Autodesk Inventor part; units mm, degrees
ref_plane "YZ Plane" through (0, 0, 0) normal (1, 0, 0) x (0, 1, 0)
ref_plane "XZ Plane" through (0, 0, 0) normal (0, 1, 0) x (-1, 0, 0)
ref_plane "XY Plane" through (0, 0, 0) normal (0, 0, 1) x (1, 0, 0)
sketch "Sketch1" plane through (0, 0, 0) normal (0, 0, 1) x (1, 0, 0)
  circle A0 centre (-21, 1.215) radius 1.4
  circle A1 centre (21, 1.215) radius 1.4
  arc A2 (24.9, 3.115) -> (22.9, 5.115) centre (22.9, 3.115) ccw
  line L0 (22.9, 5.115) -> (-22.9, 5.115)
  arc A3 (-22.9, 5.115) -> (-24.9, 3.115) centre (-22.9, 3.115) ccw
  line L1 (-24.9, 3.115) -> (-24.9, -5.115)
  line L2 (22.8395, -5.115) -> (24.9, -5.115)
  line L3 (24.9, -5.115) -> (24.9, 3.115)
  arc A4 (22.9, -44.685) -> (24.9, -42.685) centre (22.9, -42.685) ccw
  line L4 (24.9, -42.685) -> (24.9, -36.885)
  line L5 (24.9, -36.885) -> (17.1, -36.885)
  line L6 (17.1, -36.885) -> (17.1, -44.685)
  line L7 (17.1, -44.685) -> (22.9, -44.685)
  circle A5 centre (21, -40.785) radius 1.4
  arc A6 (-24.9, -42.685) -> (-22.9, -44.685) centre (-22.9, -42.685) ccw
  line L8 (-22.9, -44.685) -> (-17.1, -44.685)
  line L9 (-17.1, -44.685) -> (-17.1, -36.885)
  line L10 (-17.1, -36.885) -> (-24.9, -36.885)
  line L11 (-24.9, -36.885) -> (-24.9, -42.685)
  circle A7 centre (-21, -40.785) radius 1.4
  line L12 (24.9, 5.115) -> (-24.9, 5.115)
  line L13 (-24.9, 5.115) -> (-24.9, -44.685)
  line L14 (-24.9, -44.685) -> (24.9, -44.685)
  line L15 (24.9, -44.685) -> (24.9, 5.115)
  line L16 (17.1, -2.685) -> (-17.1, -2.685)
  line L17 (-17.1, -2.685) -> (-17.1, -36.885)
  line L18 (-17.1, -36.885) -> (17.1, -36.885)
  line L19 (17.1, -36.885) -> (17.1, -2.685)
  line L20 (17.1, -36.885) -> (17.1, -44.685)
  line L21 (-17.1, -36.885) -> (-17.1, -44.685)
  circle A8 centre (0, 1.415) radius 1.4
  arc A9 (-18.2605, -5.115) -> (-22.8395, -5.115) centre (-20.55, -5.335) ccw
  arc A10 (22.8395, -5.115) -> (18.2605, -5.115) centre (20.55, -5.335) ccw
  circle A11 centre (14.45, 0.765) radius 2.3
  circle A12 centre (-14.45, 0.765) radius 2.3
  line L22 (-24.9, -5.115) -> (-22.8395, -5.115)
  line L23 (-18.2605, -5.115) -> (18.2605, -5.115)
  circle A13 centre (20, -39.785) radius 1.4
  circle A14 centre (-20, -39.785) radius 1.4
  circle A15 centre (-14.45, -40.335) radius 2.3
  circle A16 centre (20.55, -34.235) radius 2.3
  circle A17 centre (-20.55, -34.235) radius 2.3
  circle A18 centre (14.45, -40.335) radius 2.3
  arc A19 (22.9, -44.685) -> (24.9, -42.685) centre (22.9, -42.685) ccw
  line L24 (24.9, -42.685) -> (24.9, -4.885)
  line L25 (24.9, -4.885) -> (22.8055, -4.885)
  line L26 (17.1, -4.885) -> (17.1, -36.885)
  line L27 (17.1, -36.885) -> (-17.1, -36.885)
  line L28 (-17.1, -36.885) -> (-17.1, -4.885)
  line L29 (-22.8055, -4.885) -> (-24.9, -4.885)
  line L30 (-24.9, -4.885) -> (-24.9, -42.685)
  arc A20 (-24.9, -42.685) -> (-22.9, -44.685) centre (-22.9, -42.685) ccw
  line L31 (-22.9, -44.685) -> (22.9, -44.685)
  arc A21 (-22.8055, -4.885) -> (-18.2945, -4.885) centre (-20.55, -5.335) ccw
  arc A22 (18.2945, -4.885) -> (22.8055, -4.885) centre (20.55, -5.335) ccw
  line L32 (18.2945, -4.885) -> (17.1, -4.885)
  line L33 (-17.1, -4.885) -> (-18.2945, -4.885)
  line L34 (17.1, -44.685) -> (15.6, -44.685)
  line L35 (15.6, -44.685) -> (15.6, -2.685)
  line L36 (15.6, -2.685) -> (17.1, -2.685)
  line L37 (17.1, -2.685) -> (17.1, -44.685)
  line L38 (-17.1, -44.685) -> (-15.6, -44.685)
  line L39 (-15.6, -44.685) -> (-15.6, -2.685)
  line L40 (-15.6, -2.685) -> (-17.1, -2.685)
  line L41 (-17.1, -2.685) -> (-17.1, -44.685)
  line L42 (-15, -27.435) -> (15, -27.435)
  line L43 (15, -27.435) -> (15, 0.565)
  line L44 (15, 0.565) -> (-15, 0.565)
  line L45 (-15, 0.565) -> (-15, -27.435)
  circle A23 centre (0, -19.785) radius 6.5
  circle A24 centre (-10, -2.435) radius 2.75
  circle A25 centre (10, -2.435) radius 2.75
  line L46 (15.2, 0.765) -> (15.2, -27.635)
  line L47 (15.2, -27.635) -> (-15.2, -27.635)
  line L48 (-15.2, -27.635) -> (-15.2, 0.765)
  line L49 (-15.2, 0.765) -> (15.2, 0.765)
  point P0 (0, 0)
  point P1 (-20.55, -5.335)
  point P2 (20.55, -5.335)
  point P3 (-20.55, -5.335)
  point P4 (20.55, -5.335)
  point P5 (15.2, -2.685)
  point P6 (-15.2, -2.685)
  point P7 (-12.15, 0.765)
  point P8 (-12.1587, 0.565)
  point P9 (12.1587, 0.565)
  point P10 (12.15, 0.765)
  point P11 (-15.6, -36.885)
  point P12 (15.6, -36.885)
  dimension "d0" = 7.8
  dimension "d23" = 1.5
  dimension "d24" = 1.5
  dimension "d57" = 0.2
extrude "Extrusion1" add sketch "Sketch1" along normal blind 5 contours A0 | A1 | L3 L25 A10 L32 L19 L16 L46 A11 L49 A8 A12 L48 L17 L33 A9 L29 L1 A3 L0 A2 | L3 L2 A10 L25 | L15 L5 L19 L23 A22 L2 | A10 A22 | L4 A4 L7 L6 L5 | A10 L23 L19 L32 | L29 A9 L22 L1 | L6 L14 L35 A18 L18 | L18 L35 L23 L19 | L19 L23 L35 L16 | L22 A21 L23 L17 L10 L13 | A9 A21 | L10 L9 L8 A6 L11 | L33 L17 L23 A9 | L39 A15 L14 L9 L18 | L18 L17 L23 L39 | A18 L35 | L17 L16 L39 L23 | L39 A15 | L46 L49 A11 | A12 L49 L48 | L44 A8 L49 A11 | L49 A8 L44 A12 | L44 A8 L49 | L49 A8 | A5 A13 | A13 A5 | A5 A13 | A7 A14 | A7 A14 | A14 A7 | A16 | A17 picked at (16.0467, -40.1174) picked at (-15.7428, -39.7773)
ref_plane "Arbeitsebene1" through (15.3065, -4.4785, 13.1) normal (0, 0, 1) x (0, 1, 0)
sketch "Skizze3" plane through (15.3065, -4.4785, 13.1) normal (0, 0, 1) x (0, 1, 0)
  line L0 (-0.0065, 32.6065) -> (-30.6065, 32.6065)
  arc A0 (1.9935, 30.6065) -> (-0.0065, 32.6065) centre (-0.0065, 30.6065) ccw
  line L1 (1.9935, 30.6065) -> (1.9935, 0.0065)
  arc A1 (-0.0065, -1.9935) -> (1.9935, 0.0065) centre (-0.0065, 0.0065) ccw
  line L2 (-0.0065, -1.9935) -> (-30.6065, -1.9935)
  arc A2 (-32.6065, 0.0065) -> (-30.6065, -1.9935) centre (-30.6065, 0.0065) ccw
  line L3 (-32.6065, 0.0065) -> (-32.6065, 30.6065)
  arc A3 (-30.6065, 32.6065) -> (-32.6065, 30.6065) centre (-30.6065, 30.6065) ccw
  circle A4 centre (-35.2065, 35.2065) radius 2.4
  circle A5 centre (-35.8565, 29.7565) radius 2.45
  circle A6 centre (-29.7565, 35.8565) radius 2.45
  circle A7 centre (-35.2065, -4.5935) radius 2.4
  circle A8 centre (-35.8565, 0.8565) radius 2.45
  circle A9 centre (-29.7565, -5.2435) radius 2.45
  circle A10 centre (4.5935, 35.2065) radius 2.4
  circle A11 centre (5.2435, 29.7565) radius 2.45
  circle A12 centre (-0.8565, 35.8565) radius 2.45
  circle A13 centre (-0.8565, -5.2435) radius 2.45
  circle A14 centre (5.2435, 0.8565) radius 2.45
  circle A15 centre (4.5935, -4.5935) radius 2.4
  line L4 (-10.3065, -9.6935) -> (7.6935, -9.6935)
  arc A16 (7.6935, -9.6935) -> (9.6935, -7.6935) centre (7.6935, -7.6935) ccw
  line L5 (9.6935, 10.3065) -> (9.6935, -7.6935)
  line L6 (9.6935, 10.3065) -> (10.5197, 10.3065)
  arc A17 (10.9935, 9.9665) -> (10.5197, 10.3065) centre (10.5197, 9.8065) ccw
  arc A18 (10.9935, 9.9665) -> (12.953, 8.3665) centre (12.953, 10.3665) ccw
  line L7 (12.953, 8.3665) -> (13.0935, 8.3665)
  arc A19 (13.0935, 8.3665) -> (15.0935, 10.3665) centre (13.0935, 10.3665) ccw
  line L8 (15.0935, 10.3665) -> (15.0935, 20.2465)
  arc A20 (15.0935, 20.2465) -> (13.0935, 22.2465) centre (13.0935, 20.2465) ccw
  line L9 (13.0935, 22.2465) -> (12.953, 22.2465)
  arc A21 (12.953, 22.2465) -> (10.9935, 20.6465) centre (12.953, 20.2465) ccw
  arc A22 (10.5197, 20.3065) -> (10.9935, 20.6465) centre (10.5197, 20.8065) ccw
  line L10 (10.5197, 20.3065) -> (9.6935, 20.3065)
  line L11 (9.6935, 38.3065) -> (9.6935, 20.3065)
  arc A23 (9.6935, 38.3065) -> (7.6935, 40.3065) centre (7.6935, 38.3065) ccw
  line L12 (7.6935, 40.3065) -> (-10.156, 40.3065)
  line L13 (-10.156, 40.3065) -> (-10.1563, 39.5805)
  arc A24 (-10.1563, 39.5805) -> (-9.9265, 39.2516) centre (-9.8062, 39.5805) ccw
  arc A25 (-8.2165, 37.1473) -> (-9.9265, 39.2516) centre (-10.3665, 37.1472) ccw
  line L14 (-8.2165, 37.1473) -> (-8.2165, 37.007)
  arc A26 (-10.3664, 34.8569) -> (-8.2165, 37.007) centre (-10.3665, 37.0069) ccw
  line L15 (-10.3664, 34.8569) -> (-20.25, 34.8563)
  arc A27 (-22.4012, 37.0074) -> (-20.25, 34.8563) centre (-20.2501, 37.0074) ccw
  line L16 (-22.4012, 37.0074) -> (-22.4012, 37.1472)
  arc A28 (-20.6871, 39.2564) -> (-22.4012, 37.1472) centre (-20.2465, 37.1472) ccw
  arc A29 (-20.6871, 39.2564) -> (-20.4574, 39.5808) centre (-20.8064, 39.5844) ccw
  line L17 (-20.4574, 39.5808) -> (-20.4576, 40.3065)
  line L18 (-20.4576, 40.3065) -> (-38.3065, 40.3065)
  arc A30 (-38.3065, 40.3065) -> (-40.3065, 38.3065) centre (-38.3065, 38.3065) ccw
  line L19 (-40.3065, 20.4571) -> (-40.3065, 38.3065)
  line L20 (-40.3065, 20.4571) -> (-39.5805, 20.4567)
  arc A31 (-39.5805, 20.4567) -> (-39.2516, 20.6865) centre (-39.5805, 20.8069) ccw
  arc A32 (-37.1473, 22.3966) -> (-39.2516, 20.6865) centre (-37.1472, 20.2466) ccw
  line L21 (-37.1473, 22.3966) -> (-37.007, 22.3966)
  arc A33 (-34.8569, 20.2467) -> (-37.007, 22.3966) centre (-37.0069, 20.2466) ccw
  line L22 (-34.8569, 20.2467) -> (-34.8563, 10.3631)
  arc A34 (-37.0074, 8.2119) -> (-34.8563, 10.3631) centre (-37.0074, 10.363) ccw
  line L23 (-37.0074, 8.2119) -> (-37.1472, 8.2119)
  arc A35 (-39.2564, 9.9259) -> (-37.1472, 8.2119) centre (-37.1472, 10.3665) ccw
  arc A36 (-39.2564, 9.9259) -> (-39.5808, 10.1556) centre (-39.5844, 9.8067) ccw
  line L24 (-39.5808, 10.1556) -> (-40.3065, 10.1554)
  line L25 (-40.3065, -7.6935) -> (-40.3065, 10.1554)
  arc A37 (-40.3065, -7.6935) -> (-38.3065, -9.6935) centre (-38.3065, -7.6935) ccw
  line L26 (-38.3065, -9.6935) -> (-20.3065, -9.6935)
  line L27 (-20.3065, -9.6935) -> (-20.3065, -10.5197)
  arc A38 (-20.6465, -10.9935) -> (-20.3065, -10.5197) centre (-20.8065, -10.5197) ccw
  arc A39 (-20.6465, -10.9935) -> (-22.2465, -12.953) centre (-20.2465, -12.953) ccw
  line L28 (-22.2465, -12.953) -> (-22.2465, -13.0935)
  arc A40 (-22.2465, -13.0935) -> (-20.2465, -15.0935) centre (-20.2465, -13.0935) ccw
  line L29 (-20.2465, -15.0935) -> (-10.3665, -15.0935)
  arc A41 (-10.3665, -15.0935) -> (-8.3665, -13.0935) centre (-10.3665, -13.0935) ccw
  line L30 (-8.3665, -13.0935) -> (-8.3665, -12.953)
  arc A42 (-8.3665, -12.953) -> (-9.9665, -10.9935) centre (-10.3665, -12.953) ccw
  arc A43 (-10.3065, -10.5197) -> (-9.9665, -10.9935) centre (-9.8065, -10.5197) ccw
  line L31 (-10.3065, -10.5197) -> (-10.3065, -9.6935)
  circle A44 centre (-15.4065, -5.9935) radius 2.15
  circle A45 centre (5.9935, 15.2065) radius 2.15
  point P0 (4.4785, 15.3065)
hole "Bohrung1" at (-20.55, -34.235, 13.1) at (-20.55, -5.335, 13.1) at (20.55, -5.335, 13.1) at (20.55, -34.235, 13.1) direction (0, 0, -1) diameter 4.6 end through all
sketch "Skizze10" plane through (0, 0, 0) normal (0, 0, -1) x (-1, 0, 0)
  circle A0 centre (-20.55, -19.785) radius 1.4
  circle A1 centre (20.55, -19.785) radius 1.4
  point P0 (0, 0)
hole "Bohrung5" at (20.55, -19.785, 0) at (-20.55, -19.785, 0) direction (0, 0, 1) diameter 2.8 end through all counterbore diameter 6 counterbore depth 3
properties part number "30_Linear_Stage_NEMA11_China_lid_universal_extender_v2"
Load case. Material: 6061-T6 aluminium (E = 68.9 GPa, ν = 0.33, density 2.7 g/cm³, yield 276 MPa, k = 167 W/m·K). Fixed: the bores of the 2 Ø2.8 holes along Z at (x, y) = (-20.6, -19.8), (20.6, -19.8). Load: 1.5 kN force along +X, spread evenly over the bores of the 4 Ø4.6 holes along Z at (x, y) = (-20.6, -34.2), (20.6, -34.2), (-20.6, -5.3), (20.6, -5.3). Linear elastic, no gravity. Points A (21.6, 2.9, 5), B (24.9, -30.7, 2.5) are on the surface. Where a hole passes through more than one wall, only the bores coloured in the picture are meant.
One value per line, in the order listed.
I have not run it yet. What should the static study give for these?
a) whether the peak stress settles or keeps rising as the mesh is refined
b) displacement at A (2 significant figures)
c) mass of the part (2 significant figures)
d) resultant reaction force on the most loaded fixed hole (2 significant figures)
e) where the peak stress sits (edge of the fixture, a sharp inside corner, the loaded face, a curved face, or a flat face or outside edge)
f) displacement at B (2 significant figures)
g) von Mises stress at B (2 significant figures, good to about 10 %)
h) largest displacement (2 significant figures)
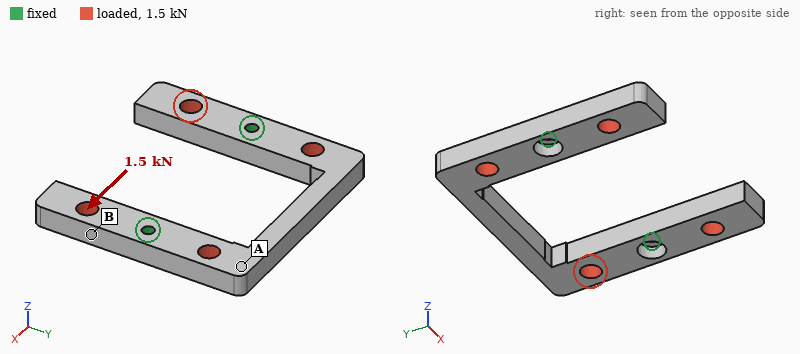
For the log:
keeps rising
29 µm
13 g
750 N
edge of the fixture
25 µm
29 MPa
62 µm
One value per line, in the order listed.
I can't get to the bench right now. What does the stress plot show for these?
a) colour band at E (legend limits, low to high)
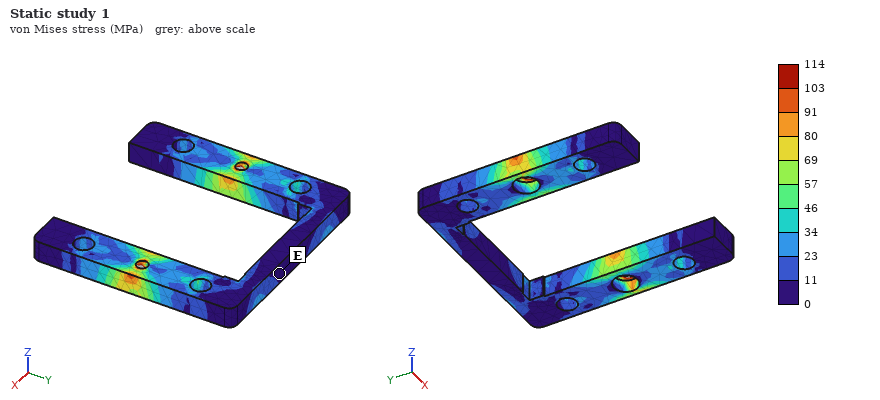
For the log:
0 to 11 MPa
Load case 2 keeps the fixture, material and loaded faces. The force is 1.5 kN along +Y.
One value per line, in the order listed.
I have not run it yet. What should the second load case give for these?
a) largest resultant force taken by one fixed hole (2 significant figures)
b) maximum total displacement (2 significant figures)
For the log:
750 N
50 µm
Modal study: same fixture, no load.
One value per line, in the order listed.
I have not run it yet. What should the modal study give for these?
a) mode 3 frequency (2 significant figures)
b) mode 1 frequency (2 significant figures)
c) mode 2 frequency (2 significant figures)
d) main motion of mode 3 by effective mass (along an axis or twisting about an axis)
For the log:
5000 Hz
2700 Hz
3900 Hz
along Z
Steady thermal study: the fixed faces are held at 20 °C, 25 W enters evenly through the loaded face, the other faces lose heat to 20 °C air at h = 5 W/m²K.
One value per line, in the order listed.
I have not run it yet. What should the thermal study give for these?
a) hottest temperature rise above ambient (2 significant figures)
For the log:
18 K
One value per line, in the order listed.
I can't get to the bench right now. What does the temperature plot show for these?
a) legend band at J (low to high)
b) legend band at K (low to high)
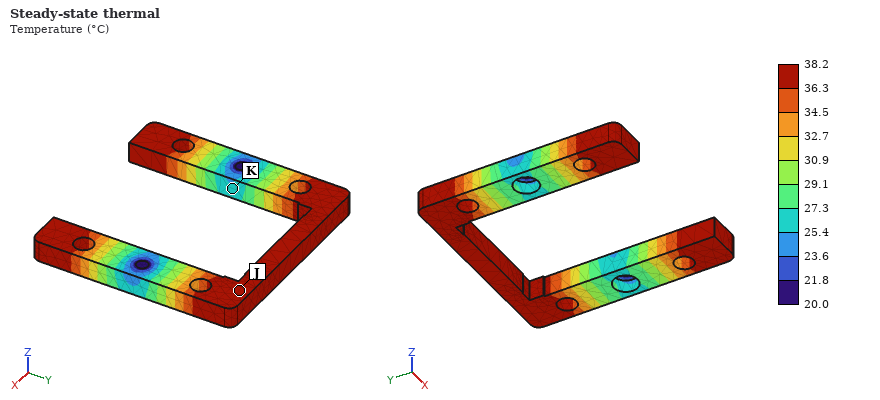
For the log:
36.3 to 38.2 °C
25.4 to 27.3 °C
